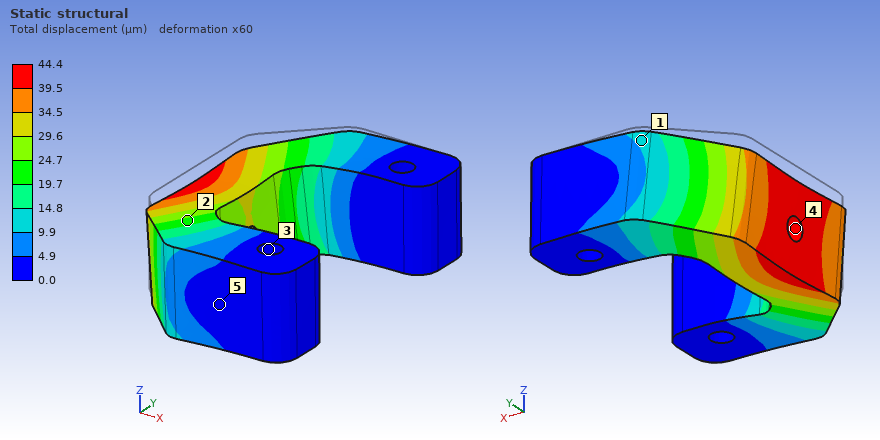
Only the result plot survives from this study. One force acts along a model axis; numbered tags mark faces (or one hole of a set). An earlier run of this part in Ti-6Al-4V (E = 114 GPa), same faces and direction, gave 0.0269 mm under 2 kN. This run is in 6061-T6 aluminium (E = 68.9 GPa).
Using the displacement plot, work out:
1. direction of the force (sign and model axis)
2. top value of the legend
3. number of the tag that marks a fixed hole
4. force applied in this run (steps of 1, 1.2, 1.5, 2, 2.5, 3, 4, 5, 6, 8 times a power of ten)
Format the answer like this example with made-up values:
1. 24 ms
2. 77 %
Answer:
1. -Z
2. 44.4 µm
3. 3
4. 2 kN
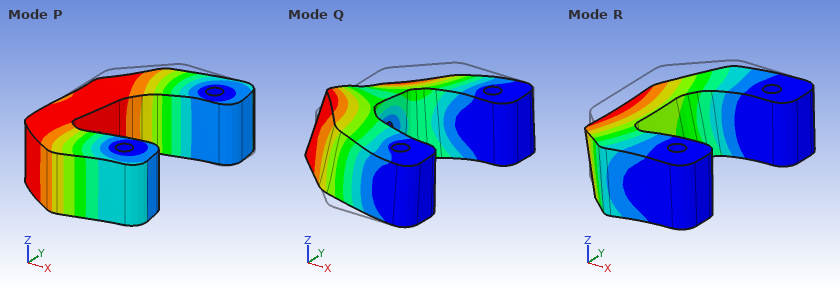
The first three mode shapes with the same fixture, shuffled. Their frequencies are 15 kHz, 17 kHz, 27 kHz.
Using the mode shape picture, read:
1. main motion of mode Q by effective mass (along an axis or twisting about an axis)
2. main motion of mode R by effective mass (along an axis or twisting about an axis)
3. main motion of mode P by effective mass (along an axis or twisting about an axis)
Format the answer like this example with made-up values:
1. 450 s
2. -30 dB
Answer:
1. twisting about X
2. along Z
3. along Y
